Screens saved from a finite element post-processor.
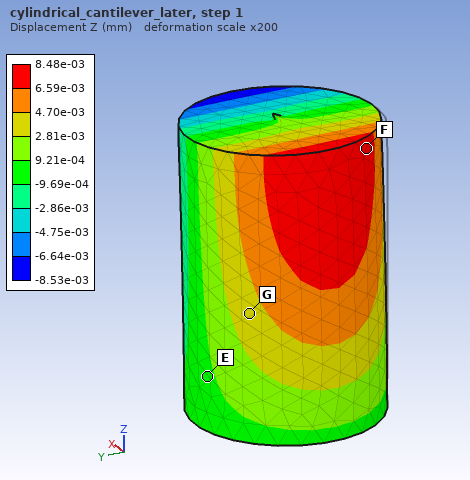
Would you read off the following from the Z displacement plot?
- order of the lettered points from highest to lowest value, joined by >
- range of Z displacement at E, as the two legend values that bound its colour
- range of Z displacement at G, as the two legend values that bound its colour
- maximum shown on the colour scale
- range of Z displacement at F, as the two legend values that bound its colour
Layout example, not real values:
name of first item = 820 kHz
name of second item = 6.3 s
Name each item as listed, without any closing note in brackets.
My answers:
order of the lettered points from highest to lowest value, joined by > = F > G > E
range of Z displacement at E, as the two legend values that bound its colour = -9.69e-04 to 9.21e-04 mm
range of Z displacement at G, as the two legend values that bound its colour = 2.81e-03 to 4.70e-03 mm
maximum shown on the colour scale = 8.48e-03 mm
range of Z displacement at F, as the two legend values that bound its colour = 6.59e-03 to 8.48e-03 mm
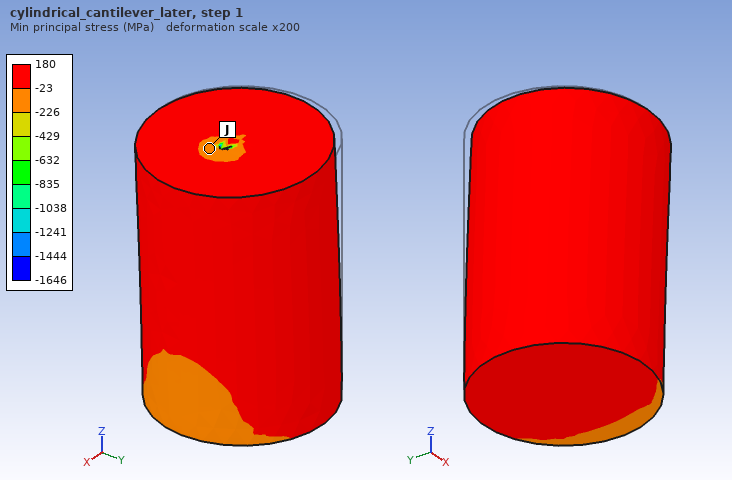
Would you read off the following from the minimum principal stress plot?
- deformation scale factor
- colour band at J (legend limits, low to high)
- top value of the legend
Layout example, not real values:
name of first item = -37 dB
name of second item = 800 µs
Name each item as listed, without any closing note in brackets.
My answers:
deformation scale factor = 200
colour band at J = -226 to -23 MPa
top value of the legend = 180 MPa
